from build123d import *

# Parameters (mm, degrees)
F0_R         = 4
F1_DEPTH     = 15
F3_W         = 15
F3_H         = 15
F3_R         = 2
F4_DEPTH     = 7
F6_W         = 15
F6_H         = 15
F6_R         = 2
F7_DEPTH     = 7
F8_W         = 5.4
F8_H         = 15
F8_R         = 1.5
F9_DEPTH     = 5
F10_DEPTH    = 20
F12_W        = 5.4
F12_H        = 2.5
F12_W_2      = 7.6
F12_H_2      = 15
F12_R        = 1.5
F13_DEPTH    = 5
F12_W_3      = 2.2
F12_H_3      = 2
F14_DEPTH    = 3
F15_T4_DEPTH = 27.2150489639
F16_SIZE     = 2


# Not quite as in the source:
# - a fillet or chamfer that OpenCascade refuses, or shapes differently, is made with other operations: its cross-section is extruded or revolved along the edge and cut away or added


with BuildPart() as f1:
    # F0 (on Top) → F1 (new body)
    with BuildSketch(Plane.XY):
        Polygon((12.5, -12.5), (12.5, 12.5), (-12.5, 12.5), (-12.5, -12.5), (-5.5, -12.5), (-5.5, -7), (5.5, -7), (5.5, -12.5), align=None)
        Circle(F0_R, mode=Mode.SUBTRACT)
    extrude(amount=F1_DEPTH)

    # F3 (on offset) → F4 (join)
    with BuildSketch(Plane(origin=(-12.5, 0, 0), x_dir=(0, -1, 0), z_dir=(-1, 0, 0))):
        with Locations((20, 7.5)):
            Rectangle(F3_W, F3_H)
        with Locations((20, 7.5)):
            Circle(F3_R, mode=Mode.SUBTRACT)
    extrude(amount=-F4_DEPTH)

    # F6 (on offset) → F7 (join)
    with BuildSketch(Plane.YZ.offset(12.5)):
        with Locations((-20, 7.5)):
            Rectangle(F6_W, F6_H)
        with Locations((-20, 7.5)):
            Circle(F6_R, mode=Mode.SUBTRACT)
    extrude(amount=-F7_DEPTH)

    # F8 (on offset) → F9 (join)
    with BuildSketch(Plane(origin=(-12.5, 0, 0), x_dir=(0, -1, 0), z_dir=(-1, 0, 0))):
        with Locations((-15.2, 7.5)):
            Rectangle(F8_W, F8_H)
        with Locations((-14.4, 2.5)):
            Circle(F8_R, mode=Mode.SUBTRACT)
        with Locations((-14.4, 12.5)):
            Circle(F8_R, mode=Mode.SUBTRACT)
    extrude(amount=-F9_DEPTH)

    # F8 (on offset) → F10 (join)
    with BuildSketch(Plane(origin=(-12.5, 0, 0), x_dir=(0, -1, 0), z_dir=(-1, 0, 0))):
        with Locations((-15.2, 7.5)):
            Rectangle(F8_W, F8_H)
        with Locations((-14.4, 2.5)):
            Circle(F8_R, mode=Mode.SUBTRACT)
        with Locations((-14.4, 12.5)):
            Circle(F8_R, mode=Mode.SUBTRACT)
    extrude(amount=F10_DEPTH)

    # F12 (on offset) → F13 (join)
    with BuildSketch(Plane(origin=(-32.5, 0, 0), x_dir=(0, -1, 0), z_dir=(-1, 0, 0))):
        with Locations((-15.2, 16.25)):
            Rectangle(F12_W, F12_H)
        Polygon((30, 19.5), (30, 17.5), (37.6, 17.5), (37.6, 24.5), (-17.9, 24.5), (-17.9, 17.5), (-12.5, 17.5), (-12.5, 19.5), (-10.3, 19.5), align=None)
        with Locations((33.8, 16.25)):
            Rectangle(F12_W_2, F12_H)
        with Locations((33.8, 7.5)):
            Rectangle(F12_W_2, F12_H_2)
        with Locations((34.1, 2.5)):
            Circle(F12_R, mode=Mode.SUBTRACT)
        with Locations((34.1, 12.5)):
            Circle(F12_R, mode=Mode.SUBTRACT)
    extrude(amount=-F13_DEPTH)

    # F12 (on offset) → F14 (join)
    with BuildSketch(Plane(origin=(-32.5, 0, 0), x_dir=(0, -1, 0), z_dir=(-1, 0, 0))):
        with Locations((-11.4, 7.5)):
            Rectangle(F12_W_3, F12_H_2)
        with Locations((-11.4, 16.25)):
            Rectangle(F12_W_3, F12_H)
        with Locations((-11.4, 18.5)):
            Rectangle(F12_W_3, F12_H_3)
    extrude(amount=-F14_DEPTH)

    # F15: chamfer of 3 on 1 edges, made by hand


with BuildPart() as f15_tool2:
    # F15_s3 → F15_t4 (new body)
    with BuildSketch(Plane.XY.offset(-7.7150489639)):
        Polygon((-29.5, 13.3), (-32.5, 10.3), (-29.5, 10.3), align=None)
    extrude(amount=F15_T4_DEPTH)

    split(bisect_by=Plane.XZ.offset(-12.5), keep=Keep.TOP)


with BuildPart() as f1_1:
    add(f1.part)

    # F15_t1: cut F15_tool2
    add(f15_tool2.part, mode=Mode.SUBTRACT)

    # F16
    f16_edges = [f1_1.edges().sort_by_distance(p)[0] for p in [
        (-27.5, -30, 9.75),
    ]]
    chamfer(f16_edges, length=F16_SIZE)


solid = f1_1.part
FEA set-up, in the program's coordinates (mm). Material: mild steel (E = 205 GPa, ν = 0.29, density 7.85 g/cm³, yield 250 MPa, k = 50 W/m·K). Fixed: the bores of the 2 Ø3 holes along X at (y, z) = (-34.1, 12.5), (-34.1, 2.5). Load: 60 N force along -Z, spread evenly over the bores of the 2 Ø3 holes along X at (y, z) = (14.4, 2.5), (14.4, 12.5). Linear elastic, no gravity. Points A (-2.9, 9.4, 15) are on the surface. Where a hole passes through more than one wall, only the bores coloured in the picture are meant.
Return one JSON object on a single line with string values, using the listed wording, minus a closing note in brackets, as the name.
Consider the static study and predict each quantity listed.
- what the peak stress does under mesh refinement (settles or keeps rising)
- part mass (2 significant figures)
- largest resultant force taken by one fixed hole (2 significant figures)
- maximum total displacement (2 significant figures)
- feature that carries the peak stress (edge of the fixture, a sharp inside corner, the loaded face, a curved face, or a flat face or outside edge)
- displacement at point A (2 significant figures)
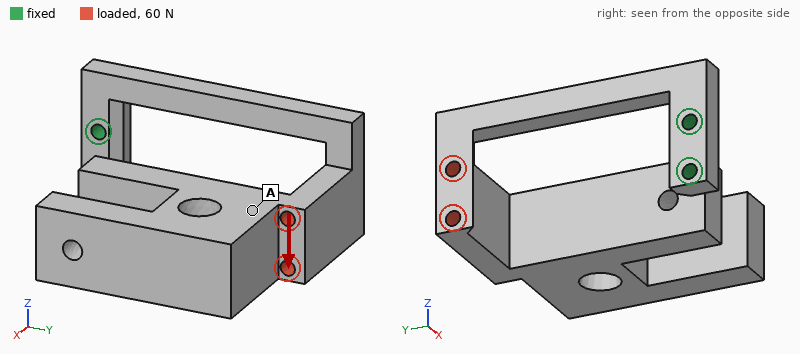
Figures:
{"what the peak stress does under mesh refinement": "keeps rising", "part mass": "110 g", "largest resultant force taken by one fixed hole": "100 N", "maximum total displacement": "0.46 mm", "feature that carries the peak stress": "a sharp inside corner", "displacement at point A": "0.33 mm"}
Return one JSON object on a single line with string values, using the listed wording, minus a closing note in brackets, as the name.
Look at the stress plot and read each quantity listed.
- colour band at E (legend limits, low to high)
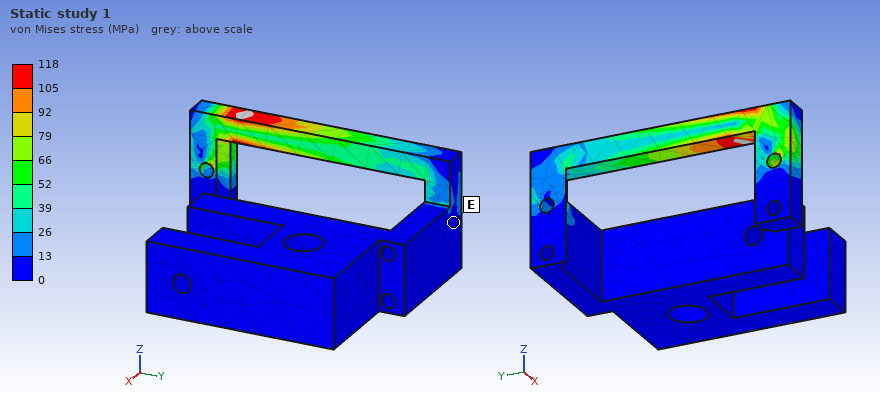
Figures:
{"colour band at E": "0 to 13 MPa"}
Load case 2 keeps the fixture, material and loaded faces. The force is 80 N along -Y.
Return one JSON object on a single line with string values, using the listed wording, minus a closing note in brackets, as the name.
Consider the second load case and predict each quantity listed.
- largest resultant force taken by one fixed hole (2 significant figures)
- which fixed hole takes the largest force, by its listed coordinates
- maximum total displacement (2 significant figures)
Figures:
{"largest resultant force taken by one fixed hole": "65 N", "which fixed hole takes the largest force, by its listed coordinates": "(-34.1, 12.5)", "maximum total displacement": "0.36 mm"}
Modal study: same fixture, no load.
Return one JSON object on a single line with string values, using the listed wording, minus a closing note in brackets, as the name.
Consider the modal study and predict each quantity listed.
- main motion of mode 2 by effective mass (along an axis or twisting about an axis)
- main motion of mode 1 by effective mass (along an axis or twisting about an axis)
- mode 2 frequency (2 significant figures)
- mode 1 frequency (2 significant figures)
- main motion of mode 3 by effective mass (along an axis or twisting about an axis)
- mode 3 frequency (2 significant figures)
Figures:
{"main motion of mode 2 by effective mass": "along Y", "main motion of mode 1 by effective mass": "along Z", "mode 2 frequency": "190 Hz", "mode 1 frequency": "160 Hz", "main motion of mode 3 by effective mass": "along X", "mode 3 frequency": "360 Hz"}
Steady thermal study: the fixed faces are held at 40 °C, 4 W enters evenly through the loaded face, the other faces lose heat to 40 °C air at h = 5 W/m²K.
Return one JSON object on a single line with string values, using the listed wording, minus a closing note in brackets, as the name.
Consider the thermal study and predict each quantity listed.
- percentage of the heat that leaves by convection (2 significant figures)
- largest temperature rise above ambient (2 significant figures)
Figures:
{"percentage of the heat that leaves by convection": "60 %", "largest temperature rise above ambient": "84 K"}
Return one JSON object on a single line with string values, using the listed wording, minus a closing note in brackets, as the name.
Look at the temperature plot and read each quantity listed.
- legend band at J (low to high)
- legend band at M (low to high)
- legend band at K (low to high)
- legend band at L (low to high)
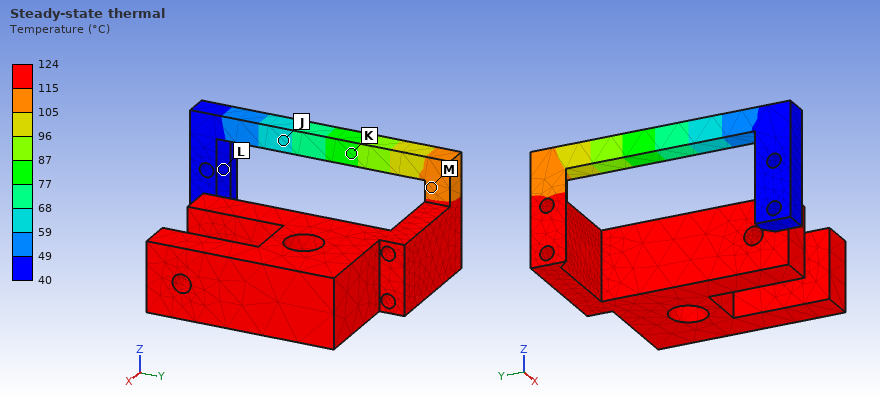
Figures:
{"legend band at J": "59 to 68 °C", "legend band at M": "105 to 115 °C", "legend band at K": "77 to 87 °C", "legend band at L": "40 to 49 °C"}
